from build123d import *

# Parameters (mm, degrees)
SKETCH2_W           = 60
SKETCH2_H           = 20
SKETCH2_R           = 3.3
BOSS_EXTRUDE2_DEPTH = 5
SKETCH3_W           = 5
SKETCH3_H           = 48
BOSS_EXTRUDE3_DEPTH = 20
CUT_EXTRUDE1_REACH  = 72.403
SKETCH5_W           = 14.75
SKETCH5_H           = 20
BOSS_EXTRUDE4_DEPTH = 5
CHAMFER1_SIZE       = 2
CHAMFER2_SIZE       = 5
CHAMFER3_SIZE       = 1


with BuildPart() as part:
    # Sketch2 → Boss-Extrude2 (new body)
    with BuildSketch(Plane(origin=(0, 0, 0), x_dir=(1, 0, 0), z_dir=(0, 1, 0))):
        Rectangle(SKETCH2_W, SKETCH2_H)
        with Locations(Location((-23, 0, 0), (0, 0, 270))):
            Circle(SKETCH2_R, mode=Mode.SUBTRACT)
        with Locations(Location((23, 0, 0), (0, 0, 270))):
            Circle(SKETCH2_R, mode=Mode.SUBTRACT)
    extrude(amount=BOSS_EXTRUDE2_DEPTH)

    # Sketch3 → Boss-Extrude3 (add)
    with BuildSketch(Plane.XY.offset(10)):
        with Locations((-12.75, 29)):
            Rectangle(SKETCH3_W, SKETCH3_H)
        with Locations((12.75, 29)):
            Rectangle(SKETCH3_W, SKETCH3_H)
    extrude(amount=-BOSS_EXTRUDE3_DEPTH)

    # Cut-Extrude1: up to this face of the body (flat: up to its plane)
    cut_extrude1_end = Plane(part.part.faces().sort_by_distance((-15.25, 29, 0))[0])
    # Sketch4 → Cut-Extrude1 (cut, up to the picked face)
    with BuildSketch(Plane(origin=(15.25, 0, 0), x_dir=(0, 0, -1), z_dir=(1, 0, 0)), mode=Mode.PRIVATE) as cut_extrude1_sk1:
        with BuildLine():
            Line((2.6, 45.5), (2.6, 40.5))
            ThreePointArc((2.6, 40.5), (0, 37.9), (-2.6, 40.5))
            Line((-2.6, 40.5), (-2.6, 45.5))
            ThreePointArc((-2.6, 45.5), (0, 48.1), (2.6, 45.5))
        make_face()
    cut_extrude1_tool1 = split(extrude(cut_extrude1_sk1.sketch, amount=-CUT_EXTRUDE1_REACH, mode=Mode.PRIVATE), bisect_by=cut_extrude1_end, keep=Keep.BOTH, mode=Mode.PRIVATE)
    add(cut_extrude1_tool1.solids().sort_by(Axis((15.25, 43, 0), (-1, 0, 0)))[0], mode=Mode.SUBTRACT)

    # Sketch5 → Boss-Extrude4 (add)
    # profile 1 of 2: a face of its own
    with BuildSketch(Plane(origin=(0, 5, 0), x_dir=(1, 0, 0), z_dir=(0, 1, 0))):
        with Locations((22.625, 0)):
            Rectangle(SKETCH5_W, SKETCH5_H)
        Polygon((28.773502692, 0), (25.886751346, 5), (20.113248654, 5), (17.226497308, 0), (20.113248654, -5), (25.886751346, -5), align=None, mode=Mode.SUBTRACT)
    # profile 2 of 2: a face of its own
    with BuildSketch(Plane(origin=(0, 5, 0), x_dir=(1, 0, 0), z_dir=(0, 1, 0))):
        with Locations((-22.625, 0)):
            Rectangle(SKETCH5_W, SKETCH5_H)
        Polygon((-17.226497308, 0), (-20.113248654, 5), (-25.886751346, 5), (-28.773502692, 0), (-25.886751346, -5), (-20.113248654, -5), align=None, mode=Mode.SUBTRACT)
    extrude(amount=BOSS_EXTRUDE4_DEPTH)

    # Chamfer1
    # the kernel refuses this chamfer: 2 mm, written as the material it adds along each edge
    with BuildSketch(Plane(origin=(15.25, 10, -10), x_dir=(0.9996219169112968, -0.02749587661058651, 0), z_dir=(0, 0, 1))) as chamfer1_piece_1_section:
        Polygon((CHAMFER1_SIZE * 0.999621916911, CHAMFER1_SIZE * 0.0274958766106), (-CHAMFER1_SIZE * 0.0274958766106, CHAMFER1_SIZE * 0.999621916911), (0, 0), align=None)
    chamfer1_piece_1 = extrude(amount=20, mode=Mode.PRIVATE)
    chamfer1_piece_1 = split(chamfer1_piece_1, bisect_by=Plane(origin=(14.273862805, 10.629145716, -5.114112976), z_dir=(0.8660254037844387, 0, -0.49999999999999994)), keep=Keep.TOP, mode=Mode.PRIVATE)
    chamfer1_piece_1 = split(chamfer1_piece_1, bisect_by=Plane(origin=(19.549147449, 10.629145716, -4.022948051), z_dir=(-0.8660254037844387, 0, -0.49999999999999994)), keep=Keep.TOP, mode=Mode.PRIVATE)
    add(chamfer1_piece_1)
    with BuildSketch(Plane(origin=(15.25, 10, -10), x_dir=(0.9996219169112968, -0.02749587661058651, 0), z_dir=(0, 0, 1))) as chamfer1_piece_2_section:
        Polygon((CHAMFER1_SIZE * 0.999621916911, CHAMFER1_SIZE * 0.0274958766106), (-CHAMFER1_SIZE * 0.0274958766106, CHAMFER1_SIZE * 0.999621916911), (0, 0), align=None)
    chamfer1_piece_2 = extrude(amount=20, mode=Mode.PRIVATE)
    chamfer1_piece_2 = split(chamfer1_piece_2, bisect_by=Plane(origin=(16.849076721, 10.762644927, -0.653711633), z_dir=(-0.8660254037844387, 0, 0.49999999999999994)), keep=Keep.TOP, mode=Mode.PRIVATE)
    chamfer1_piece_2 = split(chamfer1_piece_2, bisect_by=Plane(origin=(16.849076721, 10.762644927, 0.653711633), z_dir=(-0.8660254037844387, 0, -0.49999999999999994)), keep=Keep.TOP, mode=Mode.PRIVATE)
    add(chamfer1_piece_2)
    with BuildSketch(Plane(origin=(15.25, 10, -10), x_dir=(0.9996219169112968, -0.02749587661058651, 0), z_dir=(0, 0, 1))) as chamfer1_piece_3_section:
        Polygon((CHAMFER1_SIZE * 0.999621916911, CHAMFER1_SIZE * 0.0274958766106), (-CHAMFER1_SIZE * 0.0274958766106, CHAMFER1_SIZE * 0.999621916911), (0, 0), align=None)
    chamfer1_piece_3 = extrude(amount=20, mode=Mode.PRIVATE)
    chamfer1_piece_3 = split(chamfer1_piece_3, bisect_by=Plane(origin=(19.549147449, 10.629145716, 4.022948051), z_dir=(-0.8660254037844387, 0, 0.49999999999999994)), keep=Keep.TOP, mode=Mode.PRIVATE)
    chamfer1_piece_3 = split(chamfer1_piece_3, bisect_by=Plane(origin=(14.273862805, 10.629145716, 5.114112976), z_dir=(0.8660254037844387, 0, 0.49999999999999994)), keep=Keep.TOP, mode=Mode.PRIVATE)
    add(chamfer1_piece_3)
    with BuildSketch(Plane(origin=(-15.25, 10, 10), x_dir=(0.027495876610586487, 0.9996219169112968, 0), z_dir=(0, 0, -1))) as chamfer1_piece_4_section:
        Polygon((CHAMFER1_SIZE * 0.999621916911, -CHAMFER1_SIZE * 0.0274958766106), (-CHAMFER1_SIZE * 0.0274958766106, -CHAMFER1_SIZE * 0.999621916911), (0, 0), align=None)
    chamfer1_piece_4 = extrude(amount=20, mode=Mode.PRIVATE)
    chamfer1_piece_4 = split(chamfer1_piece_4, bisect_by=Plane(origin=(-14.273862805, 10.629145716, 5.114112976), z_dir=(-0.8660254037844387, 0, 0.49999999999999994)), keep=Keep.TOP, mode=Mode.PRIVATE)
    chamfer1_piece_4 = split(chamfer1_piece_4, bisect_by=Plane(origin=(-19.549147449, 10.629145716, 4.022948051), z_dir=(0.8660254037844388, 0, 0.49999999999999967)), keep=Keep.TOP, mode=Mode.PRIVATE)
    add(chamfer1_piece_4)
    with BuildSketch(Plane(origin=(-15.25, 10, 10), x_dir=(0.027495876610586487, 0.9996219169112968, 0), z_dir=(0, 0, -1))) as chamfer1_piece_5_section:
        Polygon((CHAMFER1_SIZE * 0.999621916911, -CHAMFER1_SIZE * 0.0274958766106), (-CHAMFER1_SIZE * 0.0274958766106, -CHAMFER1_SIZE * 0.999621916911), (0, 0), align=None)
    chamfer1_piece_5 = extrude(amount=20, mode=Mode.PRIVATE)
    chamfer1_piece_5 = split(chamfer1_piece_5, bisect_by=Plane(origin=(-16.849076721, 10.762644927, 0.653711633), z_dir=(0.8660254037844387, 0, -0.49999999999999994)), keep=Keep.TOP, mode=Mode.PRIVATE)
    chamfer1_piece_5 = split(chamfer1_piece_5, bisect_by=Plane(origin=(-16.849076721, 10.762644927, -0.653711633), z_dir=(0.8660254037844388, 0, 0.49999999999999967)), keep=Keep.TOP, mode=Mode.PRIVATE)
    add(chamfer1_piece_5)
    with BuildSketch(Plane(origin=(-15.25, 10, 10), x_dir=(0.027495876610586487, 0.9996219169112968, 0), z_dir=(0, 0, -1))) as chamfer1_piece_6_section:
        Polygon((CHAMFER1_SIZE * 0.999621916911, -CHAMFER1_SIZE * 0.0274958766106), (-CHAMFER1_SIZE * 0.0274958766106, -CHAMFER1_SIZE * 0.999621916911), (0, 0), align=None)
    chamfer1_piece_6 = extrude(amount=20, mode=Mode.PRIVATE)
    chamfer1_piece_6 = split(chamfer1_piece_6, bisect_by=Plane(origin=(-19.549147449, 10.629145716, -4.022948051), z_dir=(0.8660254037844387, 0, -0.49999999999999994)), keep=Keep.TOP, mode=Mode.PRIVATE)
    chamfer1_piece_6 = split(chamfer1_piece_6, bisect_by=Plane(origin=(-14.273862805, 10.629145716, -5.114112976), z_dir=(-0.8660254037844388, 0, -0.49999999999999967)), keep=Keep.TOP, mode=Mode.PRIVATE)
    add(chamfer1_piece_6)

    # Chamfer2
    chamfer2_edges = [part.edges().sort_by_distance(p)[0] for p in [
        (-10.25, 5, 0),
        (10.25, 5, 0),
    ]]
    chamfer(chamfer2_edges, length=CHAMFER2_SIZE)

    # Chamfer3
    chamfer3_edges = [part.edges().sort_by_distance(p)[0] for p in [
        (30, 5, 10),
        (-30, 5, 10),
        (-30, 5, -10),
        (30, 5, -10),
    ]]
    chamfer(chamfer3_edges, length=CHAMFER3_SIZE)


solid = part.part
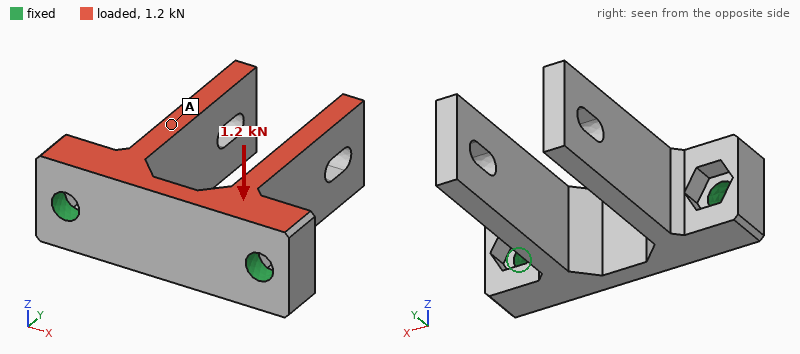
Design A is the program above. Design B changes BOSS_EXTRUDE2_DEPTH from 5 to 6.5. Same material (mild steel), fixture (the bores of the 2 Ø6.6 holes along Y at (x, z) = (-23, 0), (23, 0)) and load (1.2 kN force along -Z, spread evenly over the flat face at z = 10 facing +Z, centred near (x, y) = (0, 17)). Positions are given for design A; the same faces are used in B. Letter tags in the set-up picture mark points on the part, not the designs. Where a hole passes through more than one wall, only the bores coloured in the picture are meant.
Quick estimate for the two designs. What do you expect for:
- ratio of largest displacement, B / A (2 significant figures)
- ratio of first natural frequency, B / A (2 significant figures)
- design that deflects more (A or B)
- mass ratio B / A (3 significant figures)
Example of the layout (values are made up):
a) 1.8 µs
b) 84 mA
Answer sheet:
a) 0.73
b) 1.1
c) A
d) 1.04
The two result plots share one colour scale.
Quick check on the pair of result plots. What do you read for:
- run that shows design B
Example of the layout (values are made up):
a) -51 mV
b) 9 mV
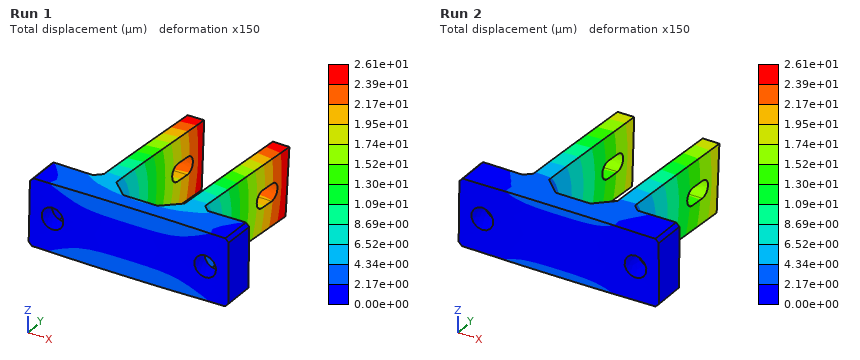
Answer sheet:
a) Run 2
